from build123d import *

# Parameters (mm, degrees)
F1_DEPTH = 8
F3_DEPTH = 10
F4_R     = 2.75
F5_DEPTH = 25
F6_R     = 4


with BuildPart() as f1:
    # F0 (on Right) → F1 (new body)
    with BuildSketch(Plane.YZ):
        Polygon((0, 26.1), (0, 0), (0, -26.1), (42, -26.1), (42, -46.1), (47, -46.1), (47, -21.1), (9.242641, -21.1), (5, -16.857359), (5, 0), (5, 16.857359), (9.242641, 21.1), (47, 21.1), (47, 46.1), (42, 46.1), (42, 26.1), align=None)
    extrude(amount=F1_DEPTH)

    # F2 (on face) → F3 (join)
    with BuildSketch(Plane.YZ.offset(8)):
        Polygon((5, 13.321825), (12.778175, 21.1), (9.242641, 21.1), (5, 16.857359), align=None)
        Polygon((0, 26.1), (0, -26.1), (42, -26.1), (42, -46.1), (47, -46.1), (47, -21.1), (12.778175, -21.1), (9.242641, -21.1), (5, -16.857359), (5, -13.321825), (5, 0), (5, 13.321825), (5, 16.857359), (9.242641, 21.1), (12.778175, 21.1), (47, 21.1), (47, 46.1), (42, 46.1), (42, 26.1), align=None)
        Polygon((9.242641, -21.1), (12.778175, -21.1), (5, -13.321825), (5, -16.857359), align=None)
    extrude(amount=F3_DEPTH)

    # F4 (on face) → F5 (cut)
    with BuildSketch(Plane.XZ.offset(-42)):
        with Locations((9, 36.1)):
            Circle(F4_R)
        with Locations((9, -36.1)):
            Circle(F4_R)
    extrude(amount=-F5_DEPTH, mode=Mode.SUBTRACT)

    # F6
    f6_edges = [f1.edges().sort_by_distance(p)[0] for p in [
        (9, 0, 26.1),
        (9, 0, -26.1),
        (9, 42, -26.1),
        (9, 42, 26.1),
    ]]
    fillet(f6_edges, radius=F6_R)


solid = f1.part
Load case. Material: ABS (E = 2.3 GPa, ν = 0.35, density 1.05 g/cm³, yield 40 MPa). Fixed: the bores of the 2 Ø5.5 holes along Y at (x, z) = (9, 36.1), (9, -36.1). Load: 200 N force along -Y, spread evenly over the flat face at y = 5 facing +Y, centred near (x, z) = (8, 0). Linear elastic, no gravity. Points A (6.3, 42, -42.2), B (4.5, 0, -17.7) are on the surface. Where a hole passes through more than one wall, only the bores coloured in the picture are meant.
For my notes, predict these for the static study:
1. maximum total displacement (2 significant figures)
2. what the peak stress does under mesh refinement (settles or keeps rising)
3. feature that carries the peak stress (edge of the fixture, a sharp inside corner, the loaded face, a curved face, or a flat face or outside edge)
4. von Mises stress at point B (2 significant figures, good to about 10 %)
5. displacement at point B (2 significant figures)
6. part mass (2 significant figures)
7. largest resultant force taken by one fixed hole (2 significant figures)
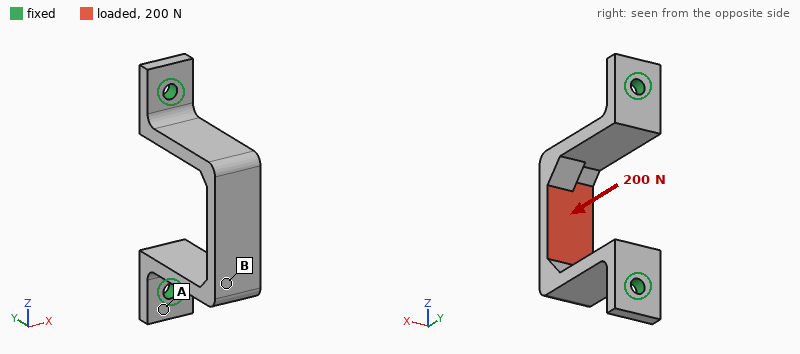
0.32 mm
keeps rising
edge of the fixture
2.1 MPa
0.14 mm
17 g
110 N
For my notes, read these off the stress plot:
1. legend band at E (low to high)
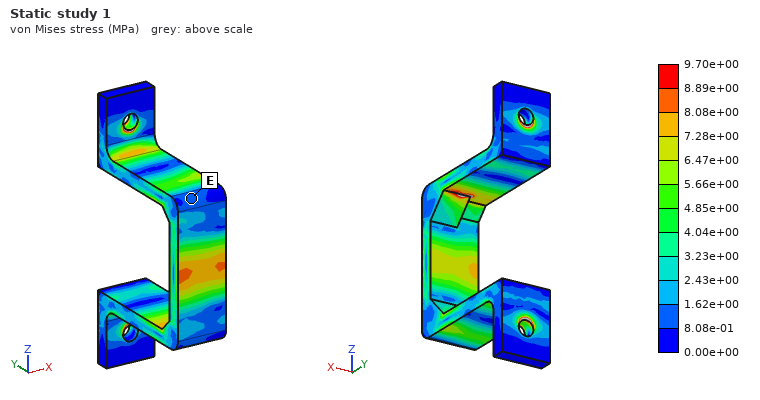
8.08e-01 to 1.62e+00 MPa
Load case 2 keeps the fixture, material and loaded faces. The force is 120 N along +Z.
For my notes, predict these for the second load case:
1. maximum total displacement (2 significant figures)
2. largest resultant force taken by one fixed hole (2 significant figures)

0.92 mm
81 N
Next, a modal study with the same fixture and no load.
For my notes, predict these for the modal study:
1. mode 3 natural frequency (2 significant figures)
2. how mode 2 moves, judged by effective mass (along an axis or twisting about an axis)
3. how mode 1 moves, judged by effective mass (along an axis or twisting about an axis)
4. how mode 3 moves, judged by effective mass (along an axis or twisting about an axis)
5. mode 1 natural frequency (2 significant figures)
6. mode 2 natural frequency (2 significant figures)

930 Hz
along Z
along X
twisting about Y
500 Hz
650 Hz
